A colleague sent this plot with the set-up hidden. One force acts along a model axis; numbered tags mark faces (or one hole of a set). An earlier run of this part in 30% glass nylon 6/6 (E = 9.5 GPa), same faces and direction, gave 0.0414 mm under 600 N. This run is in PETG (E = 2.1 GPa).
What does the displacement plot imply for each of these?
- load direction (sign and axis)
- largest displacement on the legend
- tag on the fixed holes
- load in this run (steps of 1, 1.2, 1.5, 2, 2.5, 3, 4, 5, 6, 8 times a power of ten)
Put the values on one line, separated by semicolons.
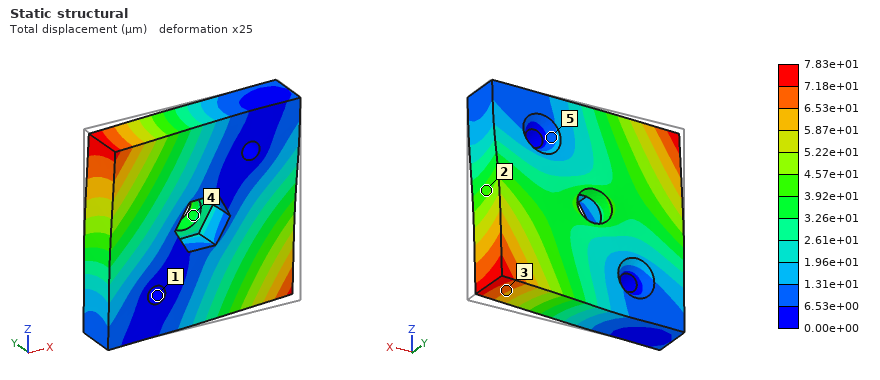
-X; 7.83e+01 µm; 1; 250 N
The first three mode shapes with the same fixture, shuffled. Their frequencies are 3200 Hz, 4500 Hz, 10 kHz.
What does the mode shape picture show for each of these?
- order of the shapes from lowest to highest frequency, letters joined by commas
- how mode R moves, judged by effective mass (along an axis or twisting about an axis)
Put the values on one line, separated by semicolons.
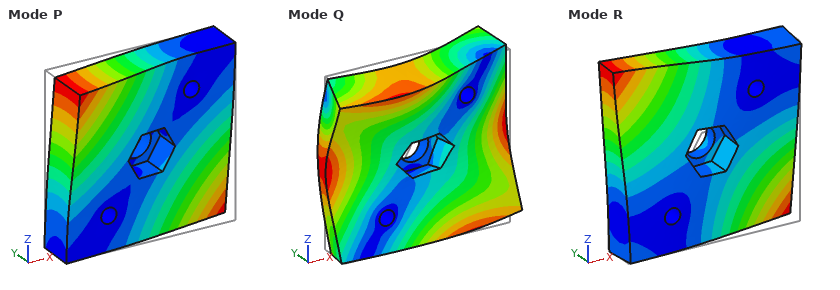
P, R, Q; along Y
